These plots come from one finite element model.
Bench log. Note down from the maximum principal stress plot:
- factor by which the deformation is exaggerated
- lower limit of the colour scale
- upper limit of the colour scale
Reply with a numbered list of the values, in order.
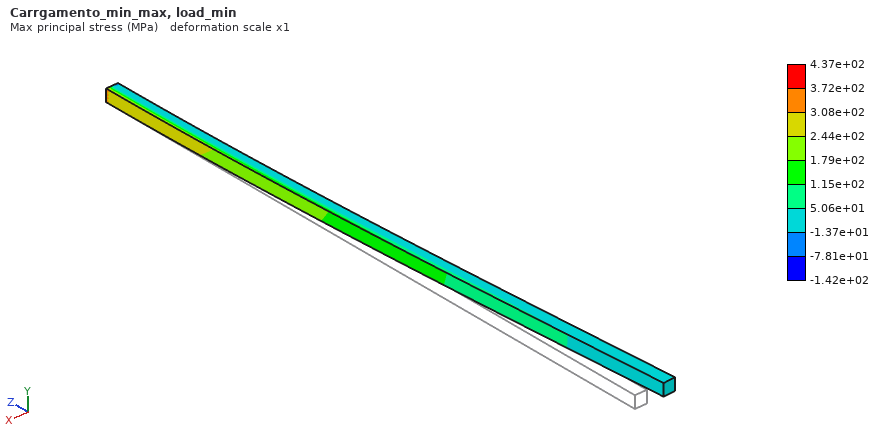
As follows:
1. 1
2. -1.42e+02 MPa
3. 4.37e+02 MPa
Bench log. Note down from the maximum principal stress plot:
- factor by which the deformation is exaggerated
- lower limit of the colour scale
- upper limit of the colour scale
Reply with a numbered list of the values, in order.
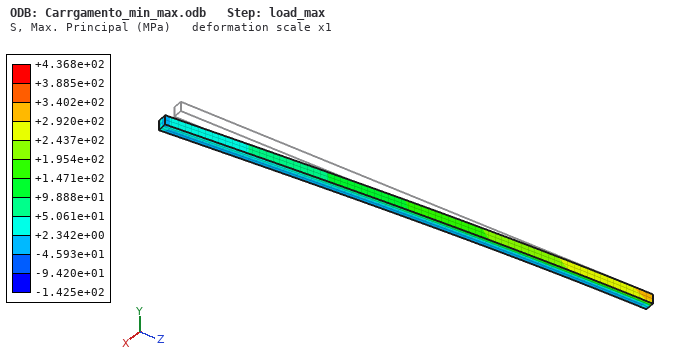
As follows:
1. 1
2. -1.425e+02 MPa
3. +4.368e+02 MPa
